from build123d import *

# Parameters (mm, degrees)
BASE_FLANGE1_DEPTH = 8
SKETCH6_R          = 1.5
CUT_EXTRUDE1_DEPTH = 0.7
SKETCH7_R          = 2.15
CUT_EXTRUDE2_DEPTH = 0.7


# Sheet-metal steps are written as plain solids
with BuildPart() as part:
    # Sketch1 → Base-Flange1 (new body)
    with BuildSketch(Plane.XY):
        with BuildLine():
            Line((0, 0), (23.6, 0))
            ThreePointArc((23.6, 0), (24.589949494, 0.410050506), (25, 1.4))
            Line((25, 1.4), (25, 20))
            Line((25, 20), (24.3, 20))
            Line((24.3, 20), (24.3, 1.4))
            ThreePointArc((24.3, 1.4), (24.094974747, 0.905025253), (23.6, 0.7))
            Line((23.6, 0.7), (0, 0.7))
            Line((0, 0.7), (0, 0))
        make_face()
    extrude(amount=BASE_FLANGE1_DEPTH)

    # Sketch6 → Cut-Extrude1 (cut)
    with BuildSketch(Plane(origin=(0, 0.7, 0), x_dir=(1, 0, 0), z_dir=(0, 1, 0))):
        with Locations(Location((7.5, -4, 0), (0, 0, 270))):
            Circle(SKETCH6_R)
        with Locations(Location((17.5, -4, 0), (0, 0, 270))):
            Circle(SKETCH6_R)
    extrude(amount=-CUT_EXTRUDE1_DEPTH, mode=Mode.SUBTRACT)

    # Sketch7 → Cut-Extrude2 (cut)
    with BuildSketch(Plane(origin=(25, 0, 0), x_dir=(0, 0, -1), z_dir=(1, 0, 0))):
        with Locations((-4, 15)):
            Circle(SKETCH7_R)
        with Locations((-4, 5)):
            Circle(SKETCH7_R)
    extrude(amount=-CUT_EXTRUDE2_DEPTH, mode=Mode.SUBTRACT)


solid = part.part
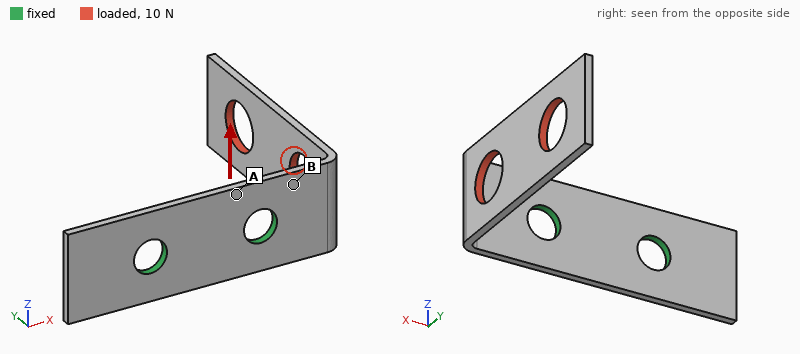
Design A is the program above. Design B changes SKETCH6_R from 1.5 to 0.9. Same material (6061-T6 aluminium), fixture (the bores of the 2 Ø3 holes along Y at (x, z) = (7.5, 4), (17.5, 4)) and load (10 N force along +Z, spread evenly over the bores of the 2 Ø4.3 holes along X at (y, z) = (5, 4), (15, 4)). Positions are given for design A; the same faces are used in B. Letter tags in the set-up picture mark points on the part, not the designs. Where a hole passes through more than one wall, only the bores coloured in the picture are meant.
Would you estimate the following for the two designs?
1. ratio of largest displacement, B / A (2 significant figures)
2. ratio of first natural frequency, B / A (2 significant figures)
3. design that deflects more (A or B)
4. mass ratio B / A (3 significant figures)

1.2
0.97
B
1.03
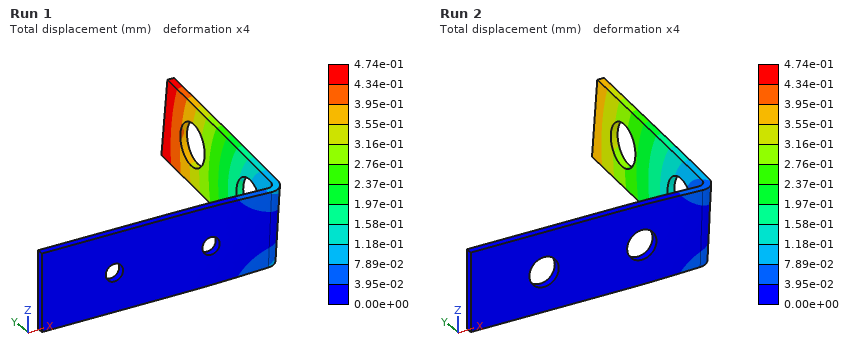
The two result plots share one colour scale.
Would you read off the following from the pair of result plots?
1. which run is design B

Run 1
